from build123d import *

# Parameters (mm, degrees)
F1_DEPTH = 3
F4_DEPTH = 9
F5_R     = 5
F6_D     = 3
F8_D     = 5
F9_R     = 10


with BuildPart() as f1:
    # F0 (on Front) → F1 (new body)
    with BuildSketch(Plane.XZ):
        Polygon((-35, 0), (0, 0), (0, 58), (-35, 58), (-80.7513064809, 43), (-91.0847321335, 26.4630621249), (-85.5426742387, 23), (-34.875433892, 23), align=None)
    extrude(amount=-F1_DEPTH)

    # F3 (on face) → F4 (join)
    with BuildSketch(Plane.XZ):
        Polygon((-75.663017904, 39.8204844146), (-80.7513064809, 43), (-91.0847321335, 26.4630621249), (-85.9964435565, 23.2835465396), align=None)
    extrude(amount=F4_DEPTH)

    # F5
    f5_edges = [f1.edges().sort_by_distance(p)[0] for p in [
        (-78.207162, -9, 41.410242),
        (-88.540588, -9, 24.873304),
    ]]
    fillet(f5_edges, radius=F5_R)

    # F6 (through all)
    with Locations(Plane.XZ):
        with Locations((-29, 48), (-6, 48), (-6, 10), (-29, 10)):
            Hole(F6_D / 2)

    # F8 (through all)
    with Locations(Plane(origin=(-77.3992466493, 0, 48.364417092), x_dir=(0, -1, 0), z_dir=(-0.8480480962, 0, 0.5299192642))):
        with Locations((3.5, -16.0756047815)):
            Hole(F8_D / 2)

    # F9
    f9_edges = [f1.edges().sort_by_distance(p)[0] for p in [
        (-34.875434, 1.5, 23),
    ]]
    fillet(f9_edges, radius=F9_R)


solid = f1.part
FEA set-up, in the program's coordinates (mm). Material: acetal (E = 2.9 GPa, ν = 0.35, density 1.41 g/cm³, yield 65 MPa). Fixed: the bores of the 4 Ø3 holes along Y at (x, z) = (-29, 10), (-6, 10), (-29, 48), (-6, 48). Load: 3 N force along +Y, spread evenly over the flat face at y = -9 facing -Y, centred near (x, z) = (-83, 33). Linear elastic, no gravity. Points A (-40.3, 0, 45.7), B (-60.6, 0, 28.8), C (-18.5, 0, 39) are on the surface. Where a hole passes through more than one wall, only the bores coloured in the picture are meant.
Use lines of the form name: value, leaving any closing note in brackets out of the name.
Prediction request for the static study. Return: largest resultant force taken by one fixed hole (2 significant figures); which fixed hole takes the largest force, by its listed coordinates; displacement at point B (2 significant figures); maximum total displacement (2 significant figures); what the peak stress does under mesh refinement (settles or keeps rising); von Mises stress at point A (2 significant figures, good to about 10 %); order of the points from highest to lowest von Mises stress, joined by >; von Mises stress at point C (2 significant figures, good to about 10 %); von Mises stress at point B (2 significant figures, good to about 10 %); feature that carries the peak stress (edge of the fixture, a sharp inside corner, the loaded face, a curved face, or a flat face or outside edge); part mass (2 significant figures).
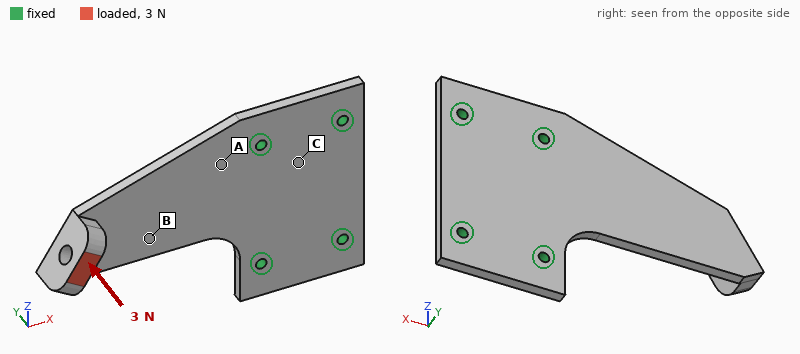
largest resultant force taken by one fixed hole: 4.4 N
which fixed hole takes the largest force, by its listed coordinates: (-29, 48)
displacement at point B: 0.35 mm
maximum total displacement: 1.0 mm
what the peak stress does under mesh refinement: keeps rising
von Mises stress at point A: 2.3 MPa
order of the points from highest to lowest von Mises stress, joined by >: A > B > C
von Mises stress at point C: 0.41 MPa
von Mises stress at point B: 1.7 MPa
feature that carries the peak stress: edge of the fixture
part mass: 16 g
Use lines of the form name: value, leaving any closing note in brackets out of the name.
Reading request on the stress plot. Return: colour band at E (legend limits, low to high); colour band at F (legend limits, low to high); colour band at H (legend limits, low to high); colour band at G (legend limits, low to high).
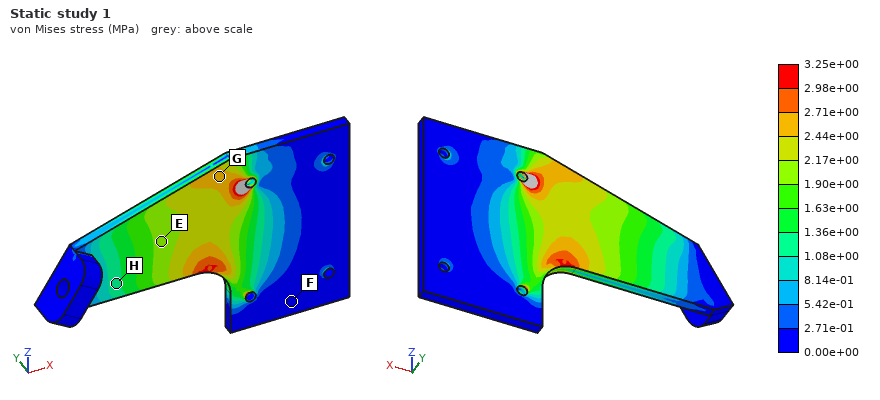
colour band at E: 1.90e+00 to 2.17e+00 MPa
colour band at F: 0.00e+00 to 2.71e-01 MPa
colour band at H: 1.08e+00 to 1.36e+00 MPa
colour band at G: 2.44e+00 to 2.71e+00 MPa
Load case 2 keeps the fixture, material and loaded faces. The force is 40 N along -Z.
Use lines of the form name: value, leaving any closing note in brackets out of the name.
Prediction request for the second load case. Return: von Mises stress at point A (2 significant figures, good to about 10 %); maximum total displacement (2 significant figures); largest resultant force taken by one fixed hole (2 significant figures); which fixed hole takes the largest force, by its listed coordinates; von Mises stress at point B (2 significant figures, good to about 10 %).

von Mises stress at point A: 5.5 MPa
maximum total displacement: 1.3 mm
largest resultant force taken by one fixed hole: 59 N
which fixed hole takes the largest force, by its listed coordinates: (-29, 48)
von Mises stress at point B: 10 MPa
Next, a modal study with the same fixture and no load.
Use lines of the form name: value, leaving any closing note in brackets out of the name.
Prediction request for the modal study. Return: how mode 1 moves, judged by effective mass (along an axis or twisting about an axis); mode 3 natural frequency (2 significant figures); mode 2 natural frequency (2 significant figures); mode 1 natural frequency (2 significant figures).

how mode 1 moves, judged by effective mass: along Y
mode 3 natural frequency: 1000 Hz
mode 2 natural frequency: 910 Hz
mode 1 natural frequency: 180 Hz
